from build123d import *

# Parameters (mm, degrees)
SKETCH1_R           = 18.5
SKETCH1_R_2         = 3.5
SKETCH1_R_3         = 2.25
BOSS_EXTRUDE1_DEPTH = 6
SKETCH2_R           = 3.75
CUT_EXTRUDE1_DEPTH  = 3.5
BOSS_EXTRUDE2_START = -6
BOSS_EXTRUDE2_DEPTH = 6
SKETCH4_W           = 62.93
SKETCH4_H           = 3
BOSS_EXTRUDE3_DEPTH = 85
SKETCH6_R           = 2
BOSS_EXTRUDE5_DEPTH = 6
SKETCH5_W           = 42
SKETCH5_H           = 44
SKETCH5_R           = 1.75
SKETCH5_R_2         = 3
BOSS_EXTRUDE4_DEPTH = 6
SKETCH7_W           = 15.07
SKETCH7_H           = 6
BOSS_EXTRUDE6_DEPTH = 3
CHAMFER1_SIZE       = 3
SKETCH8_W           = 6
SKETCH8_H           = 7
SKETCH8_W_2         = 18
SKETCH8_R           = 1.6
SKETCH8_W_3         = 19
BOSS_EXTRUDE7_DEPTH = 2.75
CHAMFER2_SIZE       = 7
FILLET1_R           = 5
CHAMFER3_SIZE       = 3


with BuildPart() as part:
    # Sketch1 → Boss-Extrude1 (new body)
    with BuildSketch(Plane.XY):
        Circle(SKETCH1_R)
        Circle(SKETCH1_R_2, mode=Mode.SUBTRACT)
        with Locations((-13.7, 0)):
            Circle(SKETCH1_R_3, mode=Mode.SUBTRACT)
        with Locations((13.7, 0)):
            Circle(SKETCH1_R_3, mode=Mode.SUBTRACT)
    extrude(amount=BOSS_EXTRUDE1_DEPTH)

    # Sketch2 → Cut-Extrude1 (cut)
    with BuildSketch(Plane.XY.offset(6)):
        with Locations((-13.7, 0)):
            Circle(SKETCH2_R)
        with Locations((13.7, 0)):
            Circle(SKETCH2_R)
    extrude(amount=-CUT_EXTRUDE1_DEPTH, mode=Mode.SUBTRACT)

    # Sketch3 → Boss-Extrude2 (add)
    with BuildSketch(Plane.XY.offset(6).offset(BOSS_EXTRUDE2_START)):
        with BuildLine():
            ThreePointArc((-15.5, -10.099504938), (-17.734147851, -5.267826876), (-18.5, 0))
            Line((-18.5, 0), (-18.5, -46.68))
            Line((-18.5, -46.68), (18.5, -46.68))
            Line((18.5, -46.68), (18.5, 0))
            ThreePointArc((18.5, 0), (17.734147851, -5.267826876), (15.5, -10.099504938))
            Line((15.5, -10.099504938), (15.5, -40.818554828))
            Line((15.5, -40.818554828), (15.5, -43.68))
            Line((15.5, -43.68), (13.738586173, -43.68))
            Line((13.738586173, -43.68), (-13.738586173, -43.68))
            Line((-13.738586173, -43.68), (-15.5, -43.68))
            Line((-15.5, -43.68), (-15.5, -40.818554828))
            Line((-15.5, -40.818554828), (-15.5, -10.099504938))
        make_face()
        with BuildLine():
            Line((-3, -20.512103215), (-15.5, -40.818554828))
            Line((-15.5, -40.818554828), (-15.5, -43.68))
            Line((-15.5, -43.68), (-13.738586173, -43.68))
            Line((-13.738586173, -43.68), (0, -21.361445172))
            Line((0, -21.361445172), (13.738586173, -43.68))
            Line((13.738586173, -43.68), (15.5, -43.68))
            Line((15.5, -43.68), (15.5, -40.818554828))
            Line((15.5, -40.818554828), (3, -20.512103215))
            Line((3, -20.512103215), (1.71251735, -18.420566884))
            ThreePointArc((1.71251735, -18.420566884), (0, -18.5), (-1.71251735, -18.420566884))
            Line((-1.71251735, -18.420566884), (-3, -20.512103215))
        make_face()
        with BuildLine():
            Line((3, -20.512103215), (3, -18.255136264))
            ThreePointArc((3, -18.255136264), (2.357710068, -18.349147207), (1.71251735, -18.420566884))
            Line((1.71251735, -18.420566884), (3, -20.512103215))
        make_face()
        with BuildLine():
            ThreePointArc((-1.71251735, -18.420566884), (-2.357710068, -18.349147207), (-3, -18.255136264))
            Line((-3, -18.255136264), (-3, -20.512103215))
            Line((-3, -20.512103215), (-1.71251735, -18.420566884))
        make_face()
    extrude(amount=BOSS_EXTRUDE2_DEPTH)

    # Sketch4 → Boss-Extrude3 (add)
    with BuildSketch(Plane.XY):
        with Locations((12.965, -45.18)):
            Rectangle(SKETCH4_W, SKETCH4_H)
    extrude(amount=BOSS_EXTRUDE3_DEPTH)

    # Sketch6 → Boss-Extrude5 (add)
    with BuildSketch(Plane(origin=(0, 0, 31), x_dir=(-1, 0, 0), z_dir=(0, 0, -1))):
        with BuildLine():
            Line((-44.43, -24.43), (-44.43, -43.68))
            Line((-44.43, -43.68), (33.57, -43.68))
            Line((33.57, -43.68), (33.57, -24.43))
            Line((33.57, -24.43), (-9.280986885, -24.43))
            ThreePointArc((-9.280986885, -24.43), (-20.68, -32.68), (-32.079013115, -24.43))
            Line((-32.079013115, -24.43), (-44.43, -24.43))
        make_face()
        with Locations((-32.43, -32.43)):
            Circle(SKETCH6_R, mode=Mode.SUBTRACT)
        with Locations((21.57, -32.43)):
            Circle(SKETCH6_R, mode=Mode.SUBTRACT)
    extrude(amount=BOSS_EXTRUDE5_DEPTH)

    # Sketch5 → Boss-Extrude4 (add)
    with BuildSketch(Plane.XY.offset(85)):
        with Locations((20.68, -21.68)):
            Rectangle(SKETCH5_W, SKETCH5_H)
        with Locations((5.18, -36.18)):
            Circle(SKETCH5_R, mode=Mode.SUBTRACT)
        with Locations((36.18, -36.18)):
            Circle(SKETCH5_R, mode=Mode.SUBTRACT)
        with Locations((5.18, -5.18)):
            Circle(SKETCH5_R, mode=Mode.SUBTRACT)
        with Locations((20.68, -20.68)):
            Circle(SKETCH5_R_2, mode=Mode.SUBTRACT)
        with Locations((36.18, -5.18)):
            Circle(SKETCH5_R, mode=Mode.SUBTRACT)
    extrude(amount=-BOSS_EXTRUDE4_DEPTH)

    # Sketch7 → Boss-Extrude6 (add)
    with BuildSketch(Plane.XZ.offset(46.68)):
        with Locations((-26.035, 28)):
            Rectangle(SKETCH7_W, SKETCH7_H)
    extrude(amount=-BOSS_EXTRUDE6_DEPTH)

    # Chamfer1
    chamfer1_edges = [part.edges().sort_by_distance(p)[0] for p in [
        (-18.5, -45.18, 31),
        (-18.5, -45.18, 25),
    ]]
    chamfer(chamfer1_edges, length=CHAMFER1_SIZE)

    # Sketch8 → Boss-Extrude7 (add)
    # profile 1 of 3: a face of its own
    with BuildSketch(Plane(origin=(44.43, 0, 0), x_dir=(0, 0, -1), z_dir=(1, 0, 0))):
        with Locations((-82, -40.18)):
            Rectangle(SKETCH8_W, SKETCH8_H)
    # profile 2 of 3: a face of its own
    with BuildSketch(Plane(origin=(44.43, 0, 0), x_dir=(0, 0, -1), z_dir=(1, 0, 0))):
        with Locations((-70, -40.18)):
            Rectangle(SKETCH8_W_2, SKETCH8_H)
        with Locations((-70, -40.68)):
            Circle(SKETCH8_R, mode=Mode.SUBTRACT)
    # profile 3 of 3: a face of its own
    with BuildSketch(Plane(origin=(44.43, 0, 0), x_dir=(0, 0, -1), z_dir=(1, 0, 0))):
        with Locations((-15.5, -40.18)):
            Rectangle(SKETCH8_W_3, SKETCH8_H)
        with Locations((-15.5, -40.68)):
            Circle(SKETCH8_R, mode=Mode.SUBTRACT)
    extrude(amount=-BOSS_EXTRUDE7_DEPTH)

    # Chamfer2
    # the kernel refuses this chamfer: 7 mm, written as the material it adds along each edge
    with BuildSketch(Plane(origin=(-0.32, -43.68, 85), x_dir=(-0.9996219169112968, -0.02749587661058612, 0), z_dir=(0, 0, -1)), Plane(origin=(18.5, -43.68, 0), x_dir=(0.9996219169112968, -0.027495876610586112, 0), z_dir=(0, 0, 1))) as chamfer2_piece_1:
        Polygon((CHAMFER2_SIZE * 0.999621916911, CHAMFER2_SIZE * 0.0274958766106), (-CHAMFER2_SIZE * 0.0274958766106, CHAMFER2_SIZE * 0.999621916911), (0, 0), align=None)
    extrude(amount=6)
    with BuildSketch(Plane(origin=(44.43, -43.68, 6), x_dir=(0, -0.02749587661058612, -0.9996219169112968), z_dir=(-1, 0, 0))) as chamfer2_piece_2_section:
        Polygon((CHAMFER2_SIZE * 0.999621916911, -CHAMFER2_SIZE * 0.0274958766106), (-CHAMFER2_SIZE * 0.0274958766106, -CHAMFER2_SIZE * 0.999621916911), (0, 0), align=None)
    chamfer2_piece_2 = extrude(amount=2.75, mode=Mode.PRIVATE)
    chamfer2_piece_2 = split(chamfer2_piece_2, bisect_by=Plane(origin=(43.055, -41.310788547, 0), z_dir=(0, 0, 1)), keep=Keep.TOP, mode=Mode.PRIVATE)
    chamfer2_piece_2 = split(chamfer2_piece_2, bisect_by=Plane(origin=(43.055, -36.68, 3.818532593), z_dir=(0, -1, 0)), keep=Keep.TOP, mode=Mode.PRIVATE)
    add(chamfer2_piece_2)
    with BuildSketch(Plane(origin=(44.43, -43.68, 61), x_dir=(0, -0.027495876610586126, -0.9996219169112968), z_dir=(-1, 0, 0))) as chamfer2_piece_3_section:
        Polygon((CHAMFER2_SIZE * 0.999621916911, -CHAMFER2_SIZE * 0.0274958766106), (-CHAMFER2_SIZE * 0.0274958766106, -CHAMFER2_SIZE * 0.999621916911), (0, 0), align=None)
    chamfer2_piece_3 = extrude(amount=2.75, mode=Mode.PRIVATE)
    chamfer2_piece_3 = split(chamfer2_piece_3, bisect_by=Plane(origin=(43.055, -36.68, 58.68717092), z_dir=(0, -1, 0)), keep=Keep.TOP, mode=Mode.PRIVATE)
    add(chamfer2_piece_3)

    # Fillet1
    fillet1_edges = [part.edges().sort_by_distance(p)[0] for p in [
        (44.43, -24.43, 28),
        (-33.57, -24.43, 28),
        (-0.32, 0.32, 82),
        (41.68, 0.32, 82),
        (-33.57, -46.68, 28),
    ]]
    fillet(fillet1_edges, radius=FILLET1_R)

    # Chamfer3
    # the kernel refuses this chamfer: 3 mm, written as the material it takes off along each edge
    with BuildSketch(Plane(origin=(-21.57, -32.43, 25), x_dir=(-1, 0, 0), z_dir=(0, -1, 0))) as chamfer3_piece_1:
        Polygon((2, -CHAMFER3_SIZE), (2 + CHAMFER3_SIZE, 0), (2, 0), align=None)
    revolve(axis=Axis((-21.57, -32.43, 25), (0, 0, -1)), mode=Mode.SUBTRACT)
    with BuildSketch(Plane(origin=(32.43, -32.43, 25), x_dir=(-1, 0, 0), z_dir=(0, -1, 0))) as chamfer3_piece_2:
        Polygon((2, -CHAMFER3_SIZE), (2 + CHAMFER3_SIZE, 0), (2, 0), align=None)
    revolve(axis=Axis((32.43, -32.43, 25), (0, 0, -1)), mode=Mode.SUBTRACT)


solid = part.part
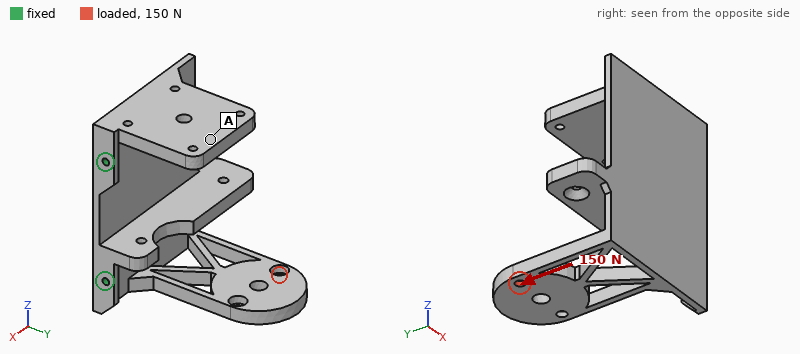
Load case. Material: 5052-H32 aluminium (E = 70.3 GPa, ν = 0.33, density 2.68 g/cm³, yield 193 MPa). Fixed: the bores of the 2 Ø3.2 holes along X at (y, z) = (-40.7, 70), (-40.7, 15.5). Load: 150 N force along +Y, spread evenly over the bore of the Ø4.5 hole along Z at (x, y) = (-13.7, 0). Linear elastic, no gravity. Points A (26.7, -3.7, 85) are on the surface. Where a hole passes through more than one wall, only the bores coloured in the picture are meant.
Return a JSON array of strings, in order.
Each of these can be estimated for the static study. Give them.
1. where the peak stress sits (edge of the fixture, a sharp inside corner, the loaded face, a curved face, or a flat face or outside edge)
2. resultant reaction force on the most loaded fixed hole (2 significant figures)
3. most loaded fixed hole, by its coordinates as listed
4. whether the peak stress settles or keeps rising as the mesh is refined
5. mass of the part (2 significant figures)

["edge of the fixture", "180 N", "(-40.7, 15.5)", "keeps rising", "120 g"]
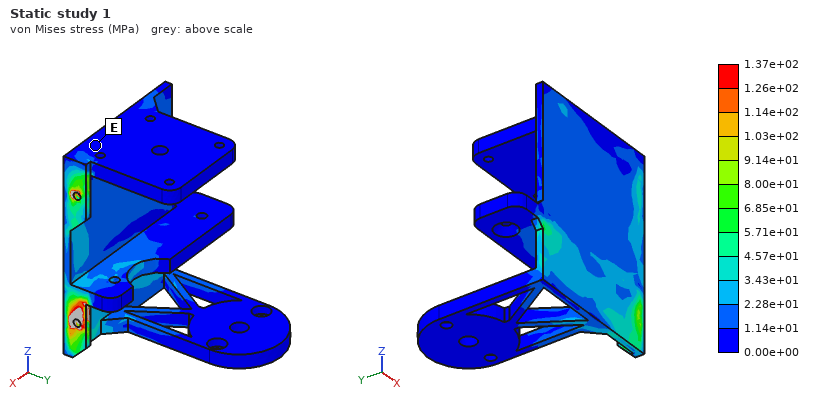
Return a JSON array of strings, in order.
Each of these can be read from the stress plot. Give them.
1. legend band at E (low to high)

["0.00e+00 to 1.14e+01 MPa"]
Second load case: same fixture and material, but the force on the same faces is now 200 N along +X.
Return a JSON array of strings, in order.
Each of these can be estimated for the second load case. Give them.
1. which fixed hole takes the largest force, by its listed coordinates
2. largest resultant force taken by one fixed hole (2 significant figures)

["(-40.7, 15.5)", "300 N"]
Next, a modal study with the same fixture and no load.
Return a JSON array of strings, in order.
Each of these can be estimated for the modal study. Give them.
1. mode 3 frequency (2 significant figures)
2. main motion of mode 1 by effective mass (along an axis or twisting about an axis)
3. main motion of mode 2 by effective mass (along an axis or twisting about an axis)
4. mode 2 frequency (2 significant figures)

["740 Hz", "along Y", "along Z", "430 Hz"]
